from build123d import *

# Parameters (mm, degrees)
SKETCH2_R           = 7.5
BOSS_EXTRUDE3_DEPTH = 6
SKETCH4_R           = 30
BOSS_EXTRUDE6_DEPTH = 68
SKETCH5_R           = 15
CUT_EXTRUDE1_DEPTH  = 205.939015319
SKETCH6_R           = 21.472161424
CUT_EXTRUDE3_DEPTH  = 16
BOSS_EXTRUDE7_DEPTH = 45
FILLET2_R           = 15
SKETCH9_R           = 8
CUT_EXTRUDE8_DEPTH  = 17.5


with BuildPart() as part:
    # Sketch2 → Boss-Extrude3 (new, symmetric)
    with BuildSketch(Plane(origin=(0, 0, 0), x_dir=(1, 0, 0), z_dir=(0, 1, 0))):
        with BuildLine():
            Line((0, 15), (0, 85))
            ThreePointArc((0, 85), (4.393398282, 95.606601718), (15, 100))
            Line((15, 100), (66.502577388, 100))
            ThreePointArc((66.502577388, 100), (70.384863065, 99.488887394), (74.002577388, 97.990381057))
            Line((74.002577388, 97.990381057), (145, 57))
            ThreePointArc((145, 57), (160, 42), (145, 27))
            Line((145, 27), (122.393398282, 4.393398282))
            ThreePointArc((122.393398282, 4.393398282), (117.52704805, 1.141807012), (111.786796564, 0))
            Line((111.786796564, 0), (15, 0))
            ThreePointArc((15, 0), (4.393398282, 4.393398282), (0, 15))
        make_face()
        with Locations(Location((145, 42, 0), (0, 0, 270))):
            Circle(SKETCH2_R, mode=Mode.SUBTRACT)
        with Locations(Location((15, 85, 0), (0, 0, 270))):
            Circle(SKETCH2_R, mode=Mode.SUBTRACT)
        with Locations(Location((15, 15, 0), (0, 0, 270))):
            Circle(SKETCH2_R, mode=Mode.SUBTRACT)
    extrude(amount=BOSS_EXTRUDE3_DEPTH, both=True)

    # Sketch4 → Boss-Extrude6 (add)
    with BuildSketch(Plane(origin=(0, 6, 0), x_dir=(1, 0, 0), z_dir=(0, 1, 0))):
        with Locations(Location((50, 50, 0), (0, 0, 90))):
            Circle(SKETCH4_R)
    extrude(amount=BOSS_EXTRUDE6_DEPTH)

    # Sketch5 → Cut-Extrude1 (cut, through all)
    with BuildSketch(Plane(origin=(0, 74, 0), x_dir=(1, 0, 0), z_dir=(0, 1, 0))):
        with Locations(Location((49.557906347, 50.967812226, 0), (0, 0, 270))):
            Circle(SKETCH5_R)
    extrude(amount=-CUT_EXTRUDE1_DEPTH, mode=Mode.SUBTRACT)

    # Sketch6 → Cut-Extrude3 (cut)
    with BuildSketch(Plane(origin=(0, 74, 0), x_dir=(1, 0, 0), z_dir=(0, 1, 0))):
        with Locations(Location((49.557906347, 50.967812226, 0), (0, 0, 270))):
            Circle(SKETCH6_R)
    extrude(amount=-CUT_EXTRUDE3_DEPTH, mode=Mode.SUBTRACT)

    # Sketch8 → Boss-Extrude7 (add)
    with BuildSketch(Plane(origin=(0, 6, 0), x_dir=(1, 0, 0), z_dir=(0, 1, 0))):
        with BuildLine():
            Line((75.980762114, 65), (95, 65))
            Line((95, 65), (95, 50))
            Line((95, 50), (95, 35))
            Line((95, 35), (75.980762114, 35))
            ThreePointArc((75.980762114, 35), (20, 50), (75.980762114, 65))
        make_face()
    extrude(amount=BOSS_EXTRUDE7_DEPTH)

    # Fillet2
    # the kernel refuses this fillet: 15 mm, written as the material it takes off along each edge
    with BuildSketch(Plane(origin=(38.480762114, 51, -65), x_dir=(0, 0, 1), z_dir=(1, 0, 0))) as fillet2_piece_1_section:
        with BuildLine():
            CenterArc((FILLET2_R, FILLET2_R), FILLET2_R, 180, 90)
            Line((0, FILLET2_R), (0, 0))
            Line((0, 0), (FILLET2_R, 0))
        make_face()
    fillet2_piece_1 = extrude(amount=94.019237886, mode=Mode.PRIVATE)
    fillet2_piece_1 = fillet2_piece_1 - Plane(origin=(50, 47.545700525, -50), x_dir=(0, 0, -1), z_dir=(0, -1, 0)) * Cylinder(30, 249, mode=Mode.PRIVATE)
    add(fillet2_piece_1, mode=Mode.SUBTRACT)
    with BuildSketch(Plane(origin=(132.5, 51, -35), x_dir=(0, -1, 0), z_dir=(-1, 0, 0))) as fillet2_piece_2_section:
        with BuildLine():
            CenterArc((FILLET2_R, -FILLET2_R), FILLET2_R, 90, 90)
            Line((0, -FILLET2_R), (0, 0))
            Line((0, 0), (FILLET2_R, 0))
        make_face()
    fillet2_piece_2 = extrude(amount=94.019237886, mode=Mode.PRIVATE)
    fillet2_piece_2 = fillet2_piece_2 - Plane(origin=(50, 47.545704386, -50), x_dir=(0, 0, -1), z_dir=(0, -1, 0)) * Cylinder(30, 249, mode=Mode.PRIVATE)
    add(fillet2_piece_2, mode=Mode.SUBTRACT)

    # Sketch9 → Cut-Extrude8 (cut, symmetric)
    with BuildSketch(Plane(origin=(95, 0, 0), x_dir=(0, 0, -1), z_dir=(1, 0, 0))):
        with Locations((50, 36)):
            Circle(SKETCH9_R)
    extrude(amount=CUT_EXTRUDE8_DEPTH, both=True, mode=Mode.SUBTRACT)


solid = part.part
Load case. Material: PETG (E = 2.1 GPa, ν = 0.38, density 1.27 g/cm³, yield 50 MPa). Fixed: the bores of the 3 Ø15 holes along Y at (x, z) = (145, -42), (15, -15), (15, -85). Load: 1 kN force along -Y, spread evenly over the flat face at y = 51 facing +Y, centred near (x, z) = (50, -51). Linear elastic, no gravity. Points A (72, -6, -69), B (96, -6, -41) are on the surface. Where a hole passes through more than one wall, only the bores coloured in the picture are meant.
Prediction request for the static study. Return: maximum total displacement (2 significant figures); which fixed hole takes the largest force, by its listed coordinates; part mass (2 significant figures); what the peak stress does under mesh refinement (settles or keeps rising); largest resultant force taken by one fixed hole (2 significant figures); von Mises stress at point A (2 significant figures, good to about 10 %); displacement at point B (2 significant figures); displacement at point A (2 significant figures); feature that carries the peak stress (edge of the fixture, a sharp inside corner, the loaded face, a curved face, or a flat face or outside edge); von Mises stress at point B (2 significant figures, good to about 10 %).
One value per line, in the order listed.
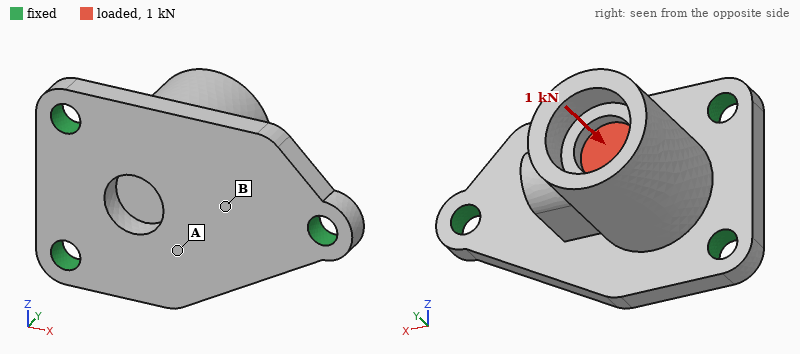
0.20 mm
(15, -85)
410 g
keeps rising
450 N
0.86 MPa
0.15 mm
0.15 mm
edge of the fixture
2.6 MPa
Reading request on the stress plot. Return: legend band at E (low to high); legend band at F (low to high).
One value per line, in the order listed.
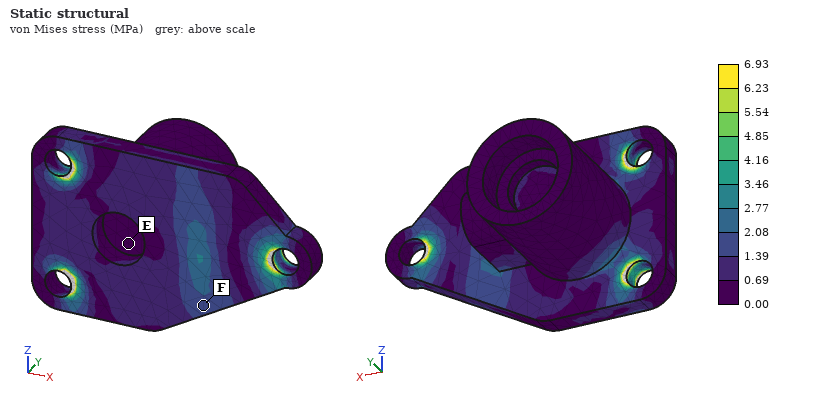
0.00 to 0.69 MPa
1.39 to 2.08 MPa
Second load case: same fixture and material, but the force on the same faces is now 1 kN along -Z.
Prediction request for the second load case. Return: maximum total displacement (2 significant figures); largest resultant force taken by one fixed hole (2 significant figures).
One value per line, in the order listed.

0.43 mm
990 N
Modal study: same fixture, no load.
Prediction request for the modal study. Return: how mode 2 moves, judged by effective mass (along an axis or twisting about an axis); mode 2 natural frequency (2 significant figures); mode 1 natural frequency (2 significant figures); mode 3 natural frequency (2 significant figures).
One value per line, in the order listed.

along Z
710 Hz
570 Hz
1300 Hz
